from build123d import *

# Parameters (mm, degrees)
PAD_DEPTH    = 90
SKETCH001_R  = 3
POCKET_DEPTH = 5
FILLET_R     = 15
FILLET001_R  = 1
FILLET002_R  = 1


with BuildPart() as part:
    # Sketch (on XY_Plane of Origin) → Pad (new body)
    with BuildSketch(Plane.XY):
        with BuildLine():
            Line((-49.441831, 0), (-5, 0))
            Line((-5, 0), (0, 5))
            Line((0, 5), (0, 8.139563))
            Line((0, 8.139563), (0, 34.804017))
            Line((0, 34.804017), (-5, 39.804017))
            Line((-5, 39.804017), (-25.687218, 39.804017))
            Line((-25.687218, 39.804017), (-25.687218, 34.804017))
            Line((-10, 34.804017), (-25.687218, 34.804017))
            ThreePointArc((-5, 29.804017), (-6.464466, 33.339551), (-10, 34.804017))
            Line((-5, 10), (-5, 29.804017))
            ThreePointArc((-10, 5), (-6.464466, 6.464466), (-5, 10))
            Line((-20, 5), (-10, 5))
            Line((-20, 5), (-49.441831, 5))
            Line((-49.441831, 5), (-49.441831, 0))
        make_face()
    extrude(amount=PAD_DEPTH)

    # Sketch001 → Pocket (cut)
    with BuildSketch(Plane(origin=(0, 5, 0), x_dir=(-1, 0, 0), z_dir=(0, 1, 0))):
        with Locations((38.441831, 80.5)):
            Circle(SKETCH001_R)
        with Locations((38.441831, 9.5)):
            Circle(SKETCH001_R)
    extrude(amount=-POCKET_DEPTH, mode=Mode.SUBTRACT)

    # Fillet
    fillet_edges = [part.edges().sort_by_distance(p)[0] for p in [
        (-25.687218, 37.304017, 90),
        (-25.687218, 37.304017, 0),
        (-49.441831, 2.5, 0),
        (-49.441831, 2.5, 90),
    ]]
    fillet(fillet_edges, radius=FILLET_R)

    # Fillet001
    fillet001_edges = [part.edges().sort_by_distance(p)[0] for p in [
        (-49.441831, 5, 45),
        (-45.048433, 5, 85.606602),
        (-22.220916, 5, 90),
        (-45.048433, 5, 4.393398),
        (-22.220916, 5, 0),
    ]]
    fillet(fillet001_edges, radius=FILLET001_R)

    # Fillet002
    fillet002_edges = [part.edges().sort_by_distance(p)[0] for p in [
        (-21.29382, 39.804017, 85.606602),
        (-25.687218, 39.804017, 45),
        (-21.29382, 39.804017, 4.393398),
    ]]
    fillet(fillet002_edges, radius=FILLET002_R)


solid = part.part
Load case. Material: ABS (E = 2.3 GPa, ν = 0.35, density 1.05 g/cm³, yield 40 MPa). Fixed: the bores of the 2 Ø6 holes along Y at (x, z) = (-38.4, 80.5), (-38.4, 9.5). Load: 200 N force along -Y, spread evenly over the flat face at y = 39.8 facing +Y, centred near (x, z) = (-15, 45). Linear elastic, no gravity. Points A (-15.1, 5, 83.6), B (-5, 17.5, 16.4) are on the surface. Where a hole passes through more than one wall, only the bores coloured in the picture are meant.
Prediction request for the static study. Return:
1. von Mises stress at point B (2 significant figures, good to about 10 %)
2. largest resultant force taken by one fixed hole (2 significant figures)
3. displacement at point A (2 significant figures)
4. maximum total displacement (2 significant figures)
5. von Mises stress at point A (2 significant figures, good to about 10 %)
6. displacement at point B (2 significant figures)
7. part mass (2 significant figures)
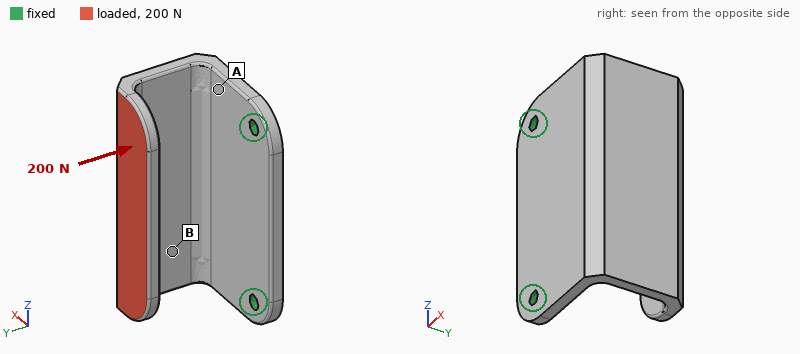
6.4 MPa
100 N
0.60 mm
1.2 mm
2.3 MPa
1.1 mm
47 g
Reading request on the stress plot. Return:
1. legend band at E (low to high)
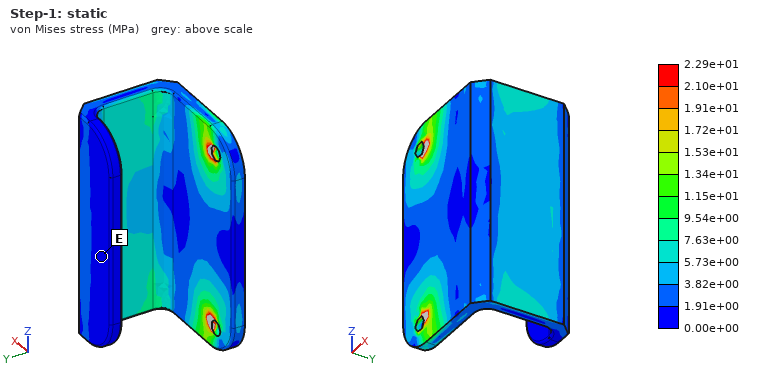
0.00e+00 to 1.91e+00 MPa
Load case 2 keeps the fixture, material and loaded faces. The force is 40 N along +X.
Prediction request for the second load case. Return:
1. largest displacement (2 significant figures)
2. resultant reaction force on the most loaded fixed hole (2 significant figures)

1.2 mm
22 N
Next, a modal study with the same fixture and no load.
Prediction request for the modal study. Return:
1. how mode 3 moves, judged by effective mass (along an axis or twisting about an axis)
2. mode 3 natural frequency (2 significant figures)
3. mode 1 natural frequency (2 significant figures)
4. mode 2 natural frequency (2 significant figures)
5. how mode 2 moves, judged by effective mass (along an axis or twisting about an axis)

along Y
530 Hz
220 Hz
400 Hz
along Z
